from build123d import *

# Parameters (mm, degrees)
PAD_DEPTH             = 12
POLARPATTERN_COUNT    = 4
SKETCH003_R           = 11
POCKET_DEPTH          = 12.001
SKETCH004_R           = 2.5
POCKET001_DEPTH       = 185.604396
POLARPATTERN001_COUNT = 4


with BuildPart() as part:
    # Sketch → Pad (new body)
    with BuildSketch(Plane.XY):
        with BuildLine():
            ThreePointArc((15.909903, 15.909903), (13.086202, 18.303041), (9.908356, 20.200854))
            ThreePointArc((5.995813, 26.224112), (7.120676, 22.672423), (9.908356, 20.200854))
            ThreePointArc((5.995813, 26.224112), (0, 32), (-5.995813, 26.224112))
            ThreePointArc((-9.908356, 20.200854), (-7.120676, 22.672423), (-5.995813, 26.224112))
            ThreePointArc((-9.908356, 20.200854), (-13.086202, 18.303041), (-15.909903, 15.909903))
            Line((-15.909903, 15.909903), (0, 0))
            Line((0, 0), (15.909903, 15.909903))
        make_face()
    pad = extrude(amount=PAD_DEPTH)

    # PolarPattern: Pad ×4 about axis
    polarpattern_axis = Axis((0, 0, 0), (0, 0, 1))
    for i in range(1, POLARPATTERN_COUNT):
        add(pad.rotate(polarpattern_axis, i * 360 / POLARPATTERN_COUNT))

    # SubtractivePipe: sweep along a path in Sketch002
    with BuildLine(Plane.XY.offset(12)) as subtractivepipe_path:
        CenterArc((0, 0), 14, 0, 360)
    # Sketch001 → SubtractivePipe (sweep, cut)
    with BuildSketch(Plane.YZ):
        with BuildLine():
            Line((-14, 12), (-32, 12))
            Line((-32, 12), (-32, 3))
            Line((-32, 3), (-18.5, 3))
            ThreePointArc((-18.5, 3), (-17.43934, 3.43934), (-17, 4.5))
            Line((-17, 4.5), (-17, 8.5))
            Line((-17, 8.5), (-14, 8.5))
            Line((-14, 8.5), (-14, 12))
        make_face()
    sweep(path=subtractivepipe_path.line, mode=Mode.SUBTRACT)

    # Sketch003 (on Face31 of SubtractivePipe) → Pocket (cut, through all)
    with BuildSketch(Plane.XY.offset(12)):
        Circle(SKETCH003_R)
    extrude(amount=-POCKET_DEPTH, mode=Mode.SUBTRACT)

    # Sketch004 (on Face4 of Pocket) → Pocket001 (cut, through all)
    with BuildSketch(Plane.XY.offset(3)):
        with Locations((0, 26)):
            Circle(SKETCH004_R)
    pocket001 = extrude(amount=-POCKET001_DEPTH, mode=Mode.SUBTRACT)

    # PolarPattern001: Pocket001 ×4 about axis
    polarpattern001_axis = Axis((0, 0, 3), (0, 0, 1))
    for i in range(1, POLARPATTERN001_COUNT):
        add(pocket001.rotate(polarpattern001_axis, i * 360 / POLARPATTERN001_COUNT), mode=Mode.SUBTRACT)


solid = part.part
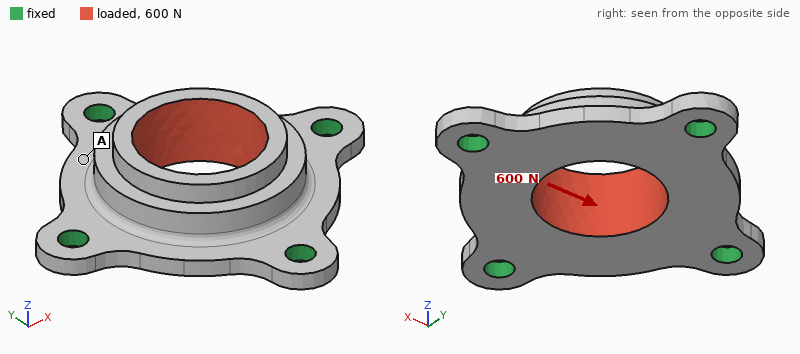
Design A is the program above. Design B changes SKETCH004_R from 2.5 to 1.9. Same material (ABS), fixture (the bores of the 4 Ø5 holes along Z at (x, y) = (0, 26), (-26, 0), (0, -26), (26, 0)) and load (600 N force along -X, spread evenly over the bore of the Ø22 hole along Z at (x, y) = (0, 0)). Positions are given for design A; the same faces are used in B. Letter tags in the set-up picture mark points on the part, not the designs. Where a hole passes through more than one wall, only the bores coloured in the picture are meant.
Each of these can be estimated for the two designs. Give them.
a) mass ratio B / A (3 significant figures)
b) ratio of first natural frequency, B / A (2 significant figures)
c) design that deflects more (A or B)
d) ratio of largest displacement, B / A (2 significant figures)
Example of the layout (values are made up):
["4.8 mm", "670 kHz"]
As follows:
["1.01", "0.90", "B", "1.1"]
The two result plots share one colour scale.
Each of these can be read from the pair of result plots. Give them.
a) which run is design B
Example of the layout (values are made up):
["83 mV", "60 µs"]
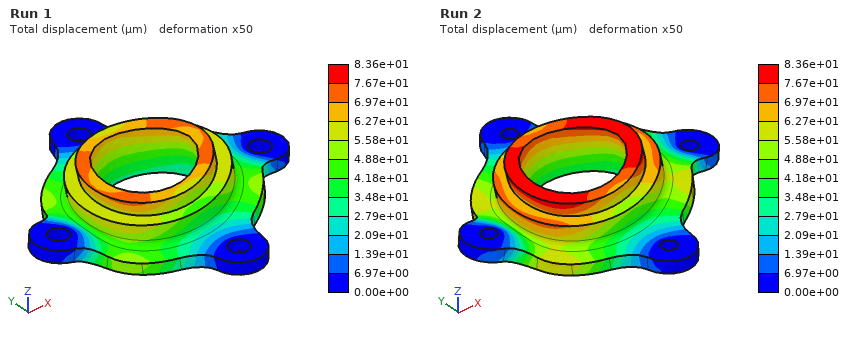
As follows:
["Run 2"]
